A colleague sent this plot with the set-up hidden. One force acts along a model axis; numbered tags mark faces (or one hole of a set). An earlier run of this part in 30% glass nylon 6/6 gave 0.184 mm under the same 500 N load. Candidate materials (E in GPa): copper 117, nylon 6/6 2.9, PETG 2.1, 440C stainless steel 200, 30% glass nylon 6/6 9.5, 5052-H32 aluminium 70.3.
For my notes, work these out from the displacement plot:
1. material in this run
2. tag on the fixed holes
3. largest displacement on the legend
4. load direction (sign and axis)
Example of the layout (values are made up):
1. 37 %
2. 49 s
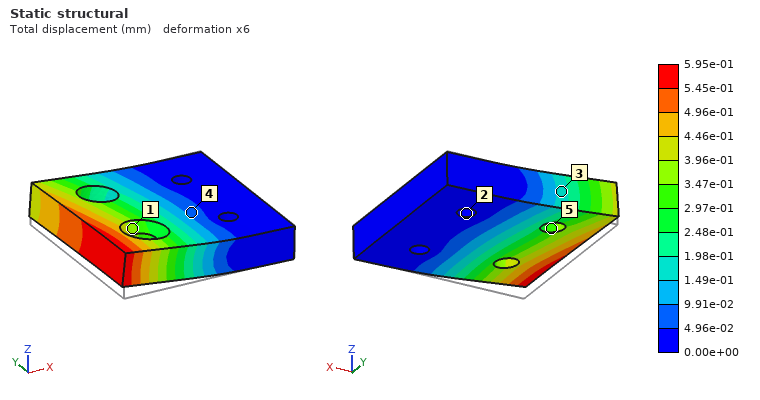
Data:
1. nylon 6/6
2. 2
3. 5.95e-01 mm
4. +Z
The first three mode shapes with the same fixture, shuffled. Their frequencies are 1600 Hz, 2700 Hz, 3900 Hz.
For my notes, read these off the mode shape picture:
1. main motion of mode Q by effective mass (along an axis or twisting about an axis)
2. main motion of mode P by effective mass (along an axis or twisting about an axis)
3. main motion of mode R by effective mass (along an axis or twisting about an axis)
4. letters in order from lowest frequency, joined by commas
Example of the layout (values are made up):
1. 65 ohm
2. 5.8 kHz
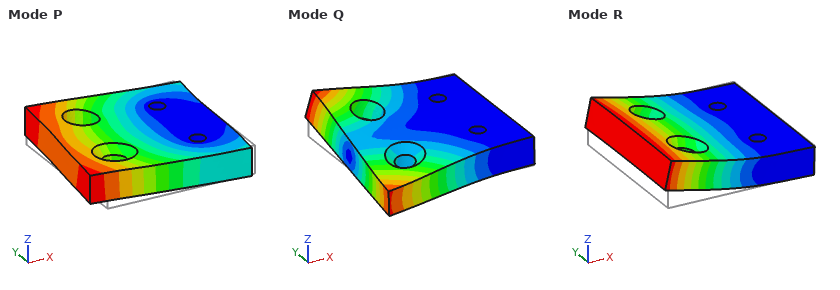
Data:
1. twisting about X
2. along Y
3. along Z
4. R, Q, P
